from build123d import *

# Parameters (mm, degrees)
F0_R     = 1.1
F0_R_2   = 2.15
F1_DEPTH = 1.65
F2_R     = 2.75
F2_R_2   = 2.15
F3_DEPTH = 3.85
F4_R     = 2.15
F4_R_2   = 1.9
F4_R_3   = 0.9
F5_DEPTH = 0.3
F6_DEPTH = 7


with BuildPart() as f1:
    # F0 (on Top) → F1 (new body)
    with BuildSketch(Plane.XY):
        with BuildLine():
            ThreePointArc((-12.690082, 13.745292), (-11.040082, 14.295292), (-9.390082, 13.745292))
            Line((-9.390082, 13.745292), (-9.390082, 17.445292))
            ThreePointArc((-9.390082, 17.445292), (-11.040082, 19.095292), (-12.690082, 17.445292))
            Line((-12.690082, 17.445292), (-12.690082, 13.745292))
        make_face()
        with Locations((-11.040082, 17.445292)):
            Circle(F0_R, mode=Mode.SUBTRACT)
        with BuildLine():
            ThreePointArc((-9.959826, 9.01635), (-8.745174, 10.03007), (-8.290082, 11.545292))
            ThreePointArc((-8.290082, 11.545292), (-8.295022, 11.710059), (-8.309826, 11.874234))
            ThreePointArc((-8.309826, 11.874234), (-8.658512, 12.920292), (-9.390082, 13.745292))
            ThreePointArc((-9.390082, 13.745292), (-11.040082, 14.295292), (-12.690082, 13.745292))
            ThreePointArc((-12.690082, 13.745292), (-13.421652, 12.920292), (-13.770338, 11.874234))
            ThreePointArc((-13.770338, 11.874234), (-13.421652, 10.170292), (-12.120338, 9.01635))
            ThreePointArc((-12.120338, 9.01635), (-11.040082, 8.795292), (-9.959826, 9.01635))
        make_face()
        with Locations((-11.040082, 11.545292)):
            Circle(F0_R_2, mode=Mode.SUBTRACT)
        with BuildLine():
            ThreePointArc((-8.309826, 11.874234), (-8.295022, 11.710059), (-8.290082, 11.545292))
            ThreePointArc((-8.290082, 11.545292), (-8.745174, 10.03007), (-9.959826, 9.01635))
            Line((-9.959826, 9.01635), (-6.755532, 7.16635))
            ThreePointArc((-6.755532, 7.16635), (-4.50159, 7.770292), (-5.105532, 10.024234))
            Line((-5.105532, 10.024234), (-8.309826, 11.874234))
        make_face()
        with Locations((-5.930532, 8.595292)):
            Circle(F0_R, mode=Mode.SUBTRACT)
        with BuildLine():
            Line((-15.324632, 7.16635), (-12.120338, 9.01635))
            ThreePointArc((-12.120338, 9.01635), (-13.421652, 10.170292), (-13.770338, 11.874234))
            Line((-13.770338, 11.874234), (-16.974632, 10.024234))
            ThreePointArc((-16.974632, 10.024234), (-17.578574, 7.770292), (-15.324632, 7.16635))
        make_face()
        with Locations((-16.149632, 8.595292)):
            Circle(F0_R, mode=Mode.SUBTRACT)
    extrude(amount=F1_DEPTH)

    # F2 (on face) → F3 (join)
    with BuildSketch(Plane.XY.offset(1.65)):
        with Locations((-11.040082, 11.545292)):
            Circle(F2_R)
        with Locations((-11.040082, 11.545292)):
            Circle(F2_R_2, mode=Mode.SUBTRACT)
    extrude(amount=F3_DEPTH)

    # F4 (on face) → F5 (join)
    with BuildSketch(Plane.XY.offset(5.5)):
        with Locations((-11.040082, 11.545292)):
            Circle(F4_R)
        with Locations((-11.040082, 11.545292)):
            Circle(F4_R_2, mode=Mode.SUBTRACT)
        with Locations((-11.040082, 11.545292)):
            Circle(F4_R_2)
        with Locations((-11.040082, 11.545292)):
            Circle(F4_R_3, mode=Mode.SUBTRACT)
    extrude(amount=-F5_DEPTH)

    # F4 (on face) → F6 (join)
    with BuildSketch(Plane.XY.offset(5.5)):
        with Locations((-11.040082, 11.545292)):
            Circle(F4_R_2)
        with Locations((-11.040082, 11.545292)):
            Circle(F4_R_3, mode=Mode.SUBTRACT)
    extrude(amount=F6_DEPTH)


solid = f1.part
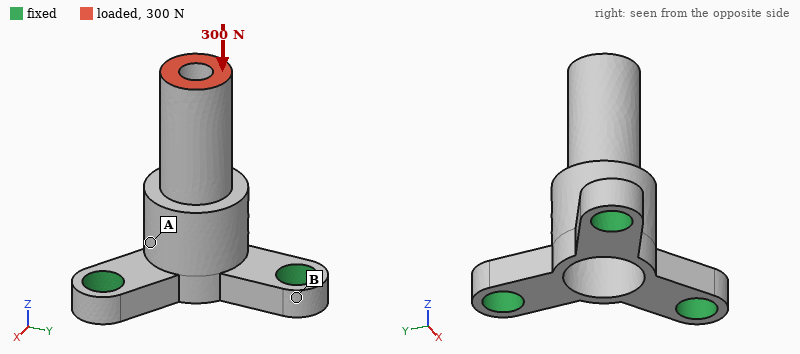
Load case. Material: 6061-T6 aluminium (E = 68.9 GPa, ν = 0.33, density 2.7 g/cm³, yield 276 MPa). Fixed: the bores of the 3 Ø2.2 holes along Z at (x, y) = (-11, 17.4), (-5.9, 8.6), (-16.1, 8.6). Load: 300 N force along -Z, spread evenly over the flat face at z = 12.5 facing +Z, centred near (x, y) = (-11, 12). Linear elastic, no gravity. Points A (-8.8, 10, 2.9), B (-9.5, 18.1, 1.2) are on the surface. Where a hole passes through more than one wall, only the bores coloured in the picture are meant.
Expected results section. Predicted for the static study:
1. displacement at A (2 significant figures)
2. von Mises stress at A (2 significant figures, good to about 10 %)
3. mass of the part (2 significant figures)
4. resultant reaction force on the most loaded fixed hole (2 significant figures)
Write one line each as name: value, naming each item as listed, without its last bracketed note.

displacement at A: 7.5 µm
von Mises stress at A: 50 MPa
mass of the part: 0.47 g
resultant reaction force on the most loaded fixed hole: 110 N
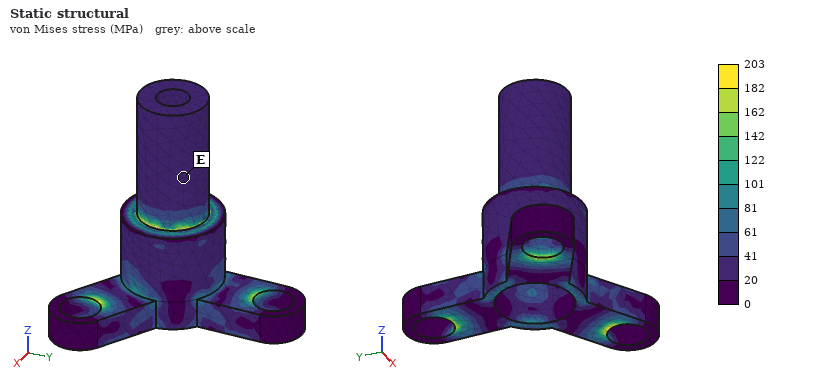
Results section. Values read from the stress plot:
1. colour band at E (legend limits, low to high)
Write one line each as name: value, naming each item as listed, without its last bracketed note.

colour band at E: 20 to 41 MPa
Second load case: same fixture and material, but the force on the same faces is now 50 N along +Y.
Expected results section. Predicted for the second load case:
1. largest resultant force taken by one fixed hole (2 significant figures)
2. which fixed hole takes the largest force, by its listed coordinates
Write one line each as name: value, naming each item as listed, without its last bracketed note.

largest resultant force taken by one fixed hole: 97 N
which fixed hole takes the largest force, by its listed coordinates: (-11, 17.4)
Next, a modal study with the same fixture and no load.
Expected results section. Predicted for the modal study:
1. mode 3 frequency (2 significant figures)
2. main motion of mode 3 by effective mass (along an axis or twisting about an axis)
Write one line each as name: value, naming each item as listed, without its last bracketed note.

mode 3 frequency: 49 kHz
main motion of mode 3 by effective mass: along Z
